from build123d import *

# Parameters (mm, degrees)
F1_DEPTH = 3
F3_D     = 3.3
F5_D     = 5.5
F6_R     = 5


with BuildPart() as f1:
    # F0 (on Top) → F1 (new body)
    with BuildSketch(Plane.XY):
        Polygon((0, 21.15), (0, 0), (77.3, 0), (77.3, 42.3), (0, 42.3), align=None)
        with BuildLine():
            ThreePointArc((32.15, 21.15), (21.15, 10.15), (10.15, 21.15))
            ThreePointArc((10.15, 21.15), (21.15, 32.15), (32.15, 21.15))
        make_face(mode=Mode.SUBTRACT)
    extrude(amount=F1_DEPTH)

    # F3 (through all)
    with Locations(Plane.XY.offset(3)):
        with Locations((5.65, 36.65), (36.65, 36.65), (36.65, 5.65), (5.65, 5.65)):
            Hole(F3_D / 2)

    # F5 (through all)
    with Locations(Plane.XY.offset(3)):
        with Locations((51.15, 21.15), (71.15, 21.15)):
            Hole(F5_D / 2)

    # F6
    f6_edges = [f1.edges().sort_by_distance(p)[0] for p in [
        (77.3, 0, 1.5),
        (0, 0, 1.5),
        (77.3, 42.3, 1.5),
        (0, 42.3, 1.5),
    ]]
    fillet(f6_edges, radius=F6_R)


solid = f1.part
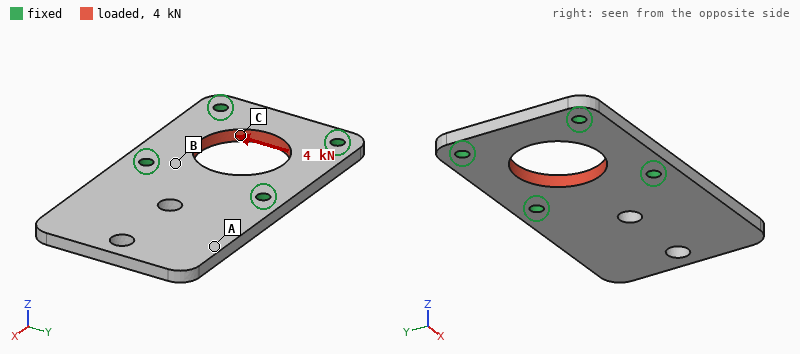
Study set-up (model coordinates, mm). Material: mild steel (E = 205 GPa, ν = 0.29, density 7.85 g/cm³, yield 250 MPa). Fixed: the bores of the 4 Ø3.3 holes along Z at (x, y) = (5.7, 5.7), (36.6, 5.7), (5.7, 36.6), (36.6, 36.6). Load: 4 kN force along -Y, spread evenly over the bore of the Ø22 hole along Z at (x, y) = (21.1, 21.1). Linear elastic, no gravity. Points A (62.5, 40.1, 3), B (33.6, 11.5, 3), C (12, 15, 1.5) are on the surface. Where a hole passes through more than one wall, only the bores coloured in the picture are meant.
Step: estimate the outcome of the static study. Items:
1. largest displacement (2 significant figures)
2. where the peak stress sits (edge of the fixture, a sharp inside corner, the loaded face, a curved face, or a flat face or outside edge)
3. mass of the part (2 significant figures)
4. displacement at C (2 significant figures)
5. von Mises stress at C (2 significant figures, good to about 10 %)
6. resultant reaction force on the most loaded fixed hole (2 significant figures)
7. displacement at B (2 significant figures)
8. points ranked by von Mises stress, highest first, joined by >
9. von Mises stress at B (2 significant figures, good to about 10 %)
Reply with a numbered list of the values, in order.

1. 3.9 µm
2. edge of the fixture
3. 66 g
4. 2.2 µm
5. 45 MPa
6. 1.0 kN
7. 1.2 µm
8. C > B > A
9. 32 MPa
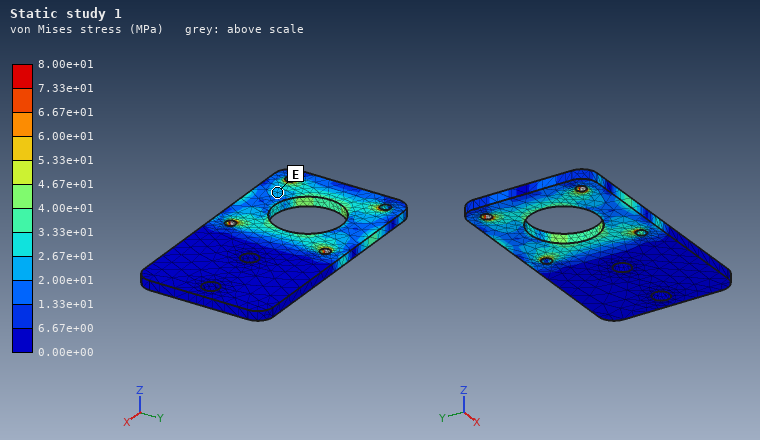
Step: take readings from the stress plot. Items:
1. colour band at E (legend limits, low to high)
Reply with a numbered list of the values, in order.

1. 2.00e+01 to 2.67e+01 MPa
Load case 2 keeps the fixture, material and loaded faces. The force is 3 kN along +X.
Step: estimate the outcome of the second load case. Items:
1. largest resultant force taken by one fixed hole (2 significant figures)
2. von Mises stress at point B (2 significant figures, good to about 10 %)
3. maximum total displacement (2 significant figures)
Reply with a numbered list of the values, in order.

1. 780 N
2. 15 MPa
3. 3.3 µm
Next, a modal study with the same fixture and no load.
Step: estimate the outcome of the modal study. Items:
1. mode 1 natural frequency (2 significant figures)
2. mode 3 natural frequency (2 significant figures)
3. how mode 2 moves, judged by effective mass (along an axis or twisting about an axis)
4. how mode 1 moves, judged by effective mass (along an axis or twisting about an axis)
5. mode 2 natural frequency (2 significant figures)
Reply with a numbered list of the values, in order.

1. 1400 Hz
2. 8700 Hz
3. twisting about X
4. along Z
5. 3600 Hz
